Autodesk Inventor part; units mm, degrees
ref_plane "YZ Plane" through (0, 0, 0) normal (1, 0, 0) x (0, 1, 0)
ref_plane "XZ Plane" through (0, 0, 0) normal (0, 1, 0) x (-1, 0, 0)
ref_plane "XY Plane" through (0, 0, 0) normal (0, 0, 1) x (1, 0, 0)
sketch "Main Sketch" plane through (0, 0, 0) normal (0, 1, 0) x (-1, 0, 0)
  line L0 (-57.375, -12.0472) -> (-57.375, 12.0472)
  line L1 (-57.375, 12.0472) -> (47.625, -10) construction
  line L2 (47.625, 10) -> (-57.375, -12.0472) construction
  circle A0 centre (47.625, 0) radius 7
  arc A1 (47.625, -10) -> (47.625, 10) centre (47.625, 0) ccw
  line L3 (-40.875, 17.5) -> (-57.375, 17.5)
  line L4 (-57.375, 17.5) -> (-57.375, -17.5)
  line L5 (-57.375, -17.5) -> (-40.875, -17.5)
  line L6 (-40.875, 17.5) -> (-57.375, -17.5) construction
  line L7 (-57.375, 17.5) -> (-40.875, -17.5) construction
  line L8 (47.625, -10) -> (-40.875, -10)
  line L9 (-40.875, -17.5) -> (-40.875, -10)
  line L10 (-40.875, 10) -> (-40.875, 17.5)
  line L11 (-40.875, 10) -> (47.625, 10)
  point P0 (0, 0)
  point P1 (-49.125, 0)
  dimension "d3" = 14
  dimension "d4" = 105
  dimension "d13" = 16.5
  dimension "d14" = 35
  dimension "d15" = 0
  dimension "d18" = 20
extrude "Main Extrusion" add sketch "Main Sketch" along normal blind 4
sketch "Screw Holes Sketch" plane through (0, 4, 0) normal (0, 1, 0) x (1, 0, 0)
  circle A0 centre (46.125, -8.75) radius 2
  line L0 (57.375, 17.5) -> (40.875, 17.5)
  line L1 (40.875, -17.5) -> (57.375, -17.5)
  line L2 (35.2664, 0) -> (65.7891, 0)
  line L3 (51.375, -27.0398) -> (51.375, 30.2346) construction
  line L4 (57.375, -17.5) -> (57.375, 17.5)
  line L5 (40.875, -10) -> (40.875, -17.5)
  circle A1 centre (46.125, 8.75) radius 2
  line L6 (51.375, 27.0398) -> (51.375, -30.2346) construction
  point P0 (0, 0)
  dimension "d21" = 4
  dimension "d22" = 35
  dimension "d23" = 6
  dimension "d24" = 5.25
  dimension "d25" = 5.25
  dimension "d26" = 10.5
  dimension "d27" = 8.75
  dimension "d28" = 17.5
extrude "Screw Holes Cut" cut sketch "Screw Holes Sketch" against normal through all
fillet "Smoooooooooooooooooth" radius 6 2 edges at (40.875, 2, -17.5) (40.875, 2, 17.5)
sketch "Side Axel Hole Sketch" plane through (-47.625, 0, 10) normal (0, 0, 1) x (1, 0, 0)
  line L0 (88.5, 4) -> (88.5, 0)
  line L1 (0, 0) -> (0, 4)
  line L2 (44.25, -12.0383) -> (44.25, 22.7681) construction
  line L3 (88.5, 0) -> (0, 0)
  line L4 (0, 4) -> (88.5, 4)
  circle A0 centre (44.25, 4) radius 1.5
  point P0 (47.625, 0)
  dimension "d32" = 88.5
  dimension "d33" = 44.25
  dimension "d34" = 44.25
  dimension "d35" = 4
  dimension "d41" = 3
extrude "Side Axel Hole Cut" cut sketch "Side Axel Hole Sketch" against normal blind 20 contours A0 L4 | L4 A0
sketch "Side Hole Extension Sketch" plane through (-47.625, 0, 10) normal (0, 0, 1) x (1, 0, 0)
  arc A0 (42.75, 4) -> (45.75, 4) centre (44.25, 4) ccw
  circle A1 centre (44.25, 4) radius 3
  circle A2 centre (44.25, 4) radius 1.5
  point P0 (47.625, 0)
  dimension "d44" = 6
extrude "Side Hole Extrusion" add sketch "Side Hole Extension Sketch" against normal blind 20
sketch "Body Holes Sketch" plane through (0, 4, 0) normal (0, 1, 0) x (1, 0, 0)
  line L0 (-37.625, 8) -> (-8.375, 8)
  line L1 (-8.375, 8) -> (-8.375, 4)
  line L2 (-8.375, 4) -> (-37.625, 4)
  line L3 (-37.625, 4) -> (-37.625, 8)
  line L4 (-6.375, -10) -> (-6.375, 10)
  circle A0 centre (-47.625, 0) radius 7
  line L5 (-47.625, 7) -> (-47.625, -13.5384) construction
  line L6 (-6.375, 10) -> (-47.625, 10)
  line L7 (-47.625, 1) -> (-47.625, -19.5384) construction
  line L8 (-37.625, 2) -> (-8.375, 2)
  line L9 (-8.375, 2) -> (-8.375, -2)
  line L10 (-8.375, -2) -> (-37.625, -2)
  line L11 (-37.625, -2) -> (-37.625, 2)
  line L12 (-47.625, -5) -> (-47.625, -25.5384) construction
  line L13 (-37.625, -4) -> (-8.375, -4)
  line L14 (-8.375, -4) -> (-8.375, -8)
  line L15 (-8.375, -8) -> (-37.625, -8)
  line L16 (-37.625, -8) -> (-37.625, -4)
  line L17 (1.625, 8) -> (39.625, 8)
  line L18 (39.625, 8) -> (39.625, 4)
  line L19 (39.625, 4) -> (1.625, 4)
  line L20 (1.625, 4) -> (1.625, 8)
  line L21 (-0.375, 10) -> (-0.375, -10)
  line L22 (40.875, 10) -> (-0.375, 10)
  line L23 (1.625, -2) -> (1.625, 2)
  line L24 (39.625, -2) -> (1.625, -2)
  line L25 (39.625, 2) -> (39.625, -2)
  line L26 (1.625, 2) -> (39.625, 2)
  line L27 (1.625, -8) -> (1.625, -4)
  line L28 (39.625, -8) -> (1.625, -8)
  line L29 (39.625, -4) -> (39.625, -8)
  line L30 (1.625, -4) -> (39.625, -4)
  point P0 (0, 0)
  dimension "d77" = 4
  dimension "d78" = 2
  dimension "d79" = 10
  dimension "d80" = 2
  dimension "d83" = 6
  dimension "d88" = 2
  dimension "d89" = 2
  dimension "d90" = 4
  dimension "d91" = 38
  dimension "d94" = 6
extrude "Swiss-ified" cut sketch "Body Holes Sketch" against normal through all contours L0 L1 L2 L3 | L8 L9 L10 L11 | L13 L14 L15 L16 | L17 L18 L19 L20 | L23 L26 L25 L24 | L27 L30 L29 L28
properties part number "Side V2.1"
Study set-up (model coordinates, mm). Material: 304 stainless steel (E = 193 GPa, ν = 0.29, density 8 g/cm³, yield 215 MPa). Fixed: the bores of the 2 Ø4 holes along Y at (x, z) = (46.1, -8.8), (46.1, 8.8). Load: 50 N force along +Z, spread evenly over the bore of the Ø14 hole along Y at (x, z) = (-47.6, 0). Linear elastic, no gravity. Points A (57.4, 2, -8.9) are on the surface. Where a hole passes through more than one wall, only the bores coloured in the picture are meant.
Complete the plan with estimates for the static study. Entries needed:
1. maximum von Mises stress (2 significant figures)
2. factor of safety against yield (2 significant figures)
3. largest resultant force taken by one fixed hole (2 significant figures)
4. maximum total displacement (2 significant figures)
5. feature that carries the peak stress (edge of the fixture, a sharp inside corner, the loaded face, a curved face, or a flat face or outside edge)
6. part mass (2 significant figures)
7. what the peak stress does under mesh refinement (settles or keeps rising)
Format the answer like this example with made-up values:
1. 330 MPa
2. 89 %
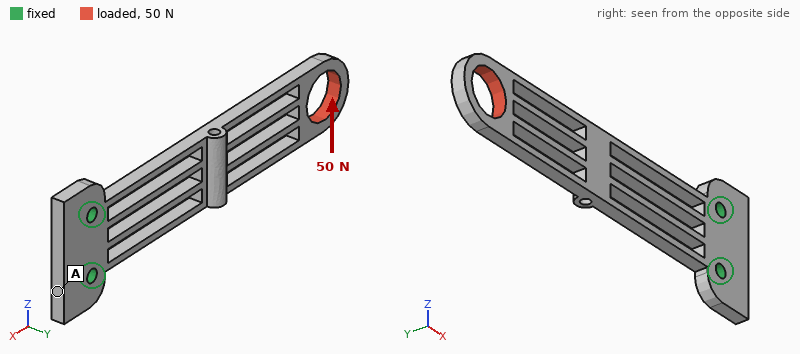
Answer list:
1. 100 MPa
2. 2.1
3. 260 N
4. 0.23 mm
5. a flat face or outside edge
6. 49 g
7. settles
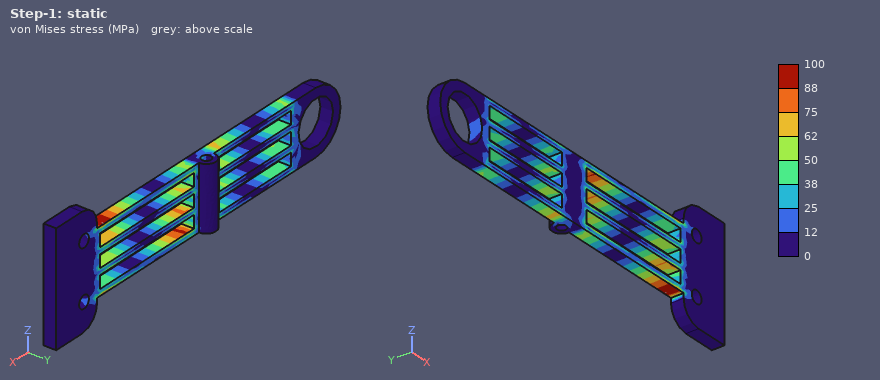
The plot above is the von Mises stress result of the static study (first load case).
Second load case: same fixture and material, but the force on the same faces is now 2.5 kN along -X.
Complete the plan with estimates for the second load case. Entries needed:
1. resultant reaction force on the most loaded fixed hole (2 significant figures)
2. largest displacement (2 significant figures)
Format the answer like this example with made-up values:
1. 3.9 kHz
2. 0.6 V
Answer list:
1. 1.3 kN
2. 50 µm
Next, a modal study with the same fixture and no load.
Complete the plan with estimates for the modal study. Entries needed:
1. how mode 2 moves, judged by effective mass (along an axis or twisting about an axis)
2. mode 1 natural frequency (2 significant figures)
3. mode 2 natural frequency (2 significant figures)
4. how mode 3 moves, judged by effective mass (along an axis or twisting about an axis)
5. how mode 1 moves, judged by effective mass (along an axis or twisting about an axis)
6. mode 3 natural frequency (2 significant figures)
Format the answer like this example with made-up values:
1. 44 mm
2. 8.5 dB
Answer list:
1. along Z
2. 290 Hz
3. 580 Hz
4. twisting about X
5. along Y
6. 1500 Hz
